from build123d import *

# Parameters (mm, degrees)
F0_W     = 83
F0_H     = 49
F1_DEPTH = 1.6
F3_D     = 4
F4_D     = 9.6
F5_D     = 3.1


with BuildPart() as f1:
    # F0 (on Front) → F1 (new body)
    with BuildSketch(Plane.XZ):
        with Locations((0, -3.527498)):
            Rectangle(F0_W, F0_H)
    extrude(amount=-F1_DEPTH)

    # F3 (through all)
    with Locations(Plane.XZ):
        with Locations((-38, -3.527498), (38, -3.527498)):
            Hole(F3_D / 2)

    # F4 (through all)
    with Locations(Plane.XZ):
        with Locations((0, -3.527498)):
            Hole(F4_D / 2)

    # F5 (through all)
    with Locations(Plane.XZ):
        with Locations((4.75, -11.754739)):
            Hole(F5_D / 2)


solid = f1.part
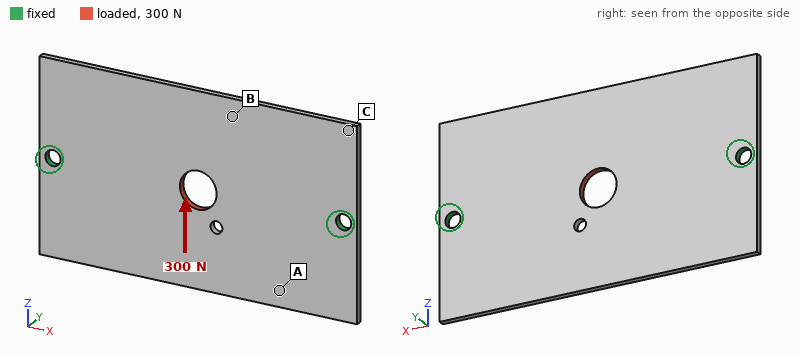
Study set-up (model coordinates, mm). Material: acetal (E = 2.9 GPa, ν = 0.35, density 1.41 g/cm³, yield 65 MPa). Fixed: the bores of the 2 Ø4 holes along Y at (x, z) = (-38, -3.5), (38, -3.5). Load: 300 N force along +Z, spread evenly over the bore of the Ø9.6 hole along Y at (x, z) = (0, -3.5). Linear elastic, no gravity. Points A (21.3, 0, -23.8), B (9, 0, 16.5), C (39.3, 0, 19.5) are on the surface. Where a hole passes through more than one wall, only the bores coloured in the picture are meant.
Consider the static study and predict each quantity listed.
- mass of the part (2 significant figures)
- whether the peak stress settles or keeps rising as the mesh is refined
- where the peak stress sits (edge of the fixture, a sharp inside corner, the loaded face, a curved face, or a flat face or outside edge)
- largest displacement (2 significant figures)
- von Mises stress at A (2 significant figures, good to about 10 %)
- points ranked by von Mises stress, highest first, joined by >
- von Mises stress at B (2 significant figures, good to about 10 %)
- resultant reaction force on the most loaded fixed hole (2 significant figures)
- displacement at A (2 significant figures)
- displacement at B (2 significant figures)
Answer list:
8.9 g
keeps rising
edge of the fixture
0.15 mm
3.6 MPa
B > A > C
6.0 MPa
150 N
0.085 mm
0.12 mm
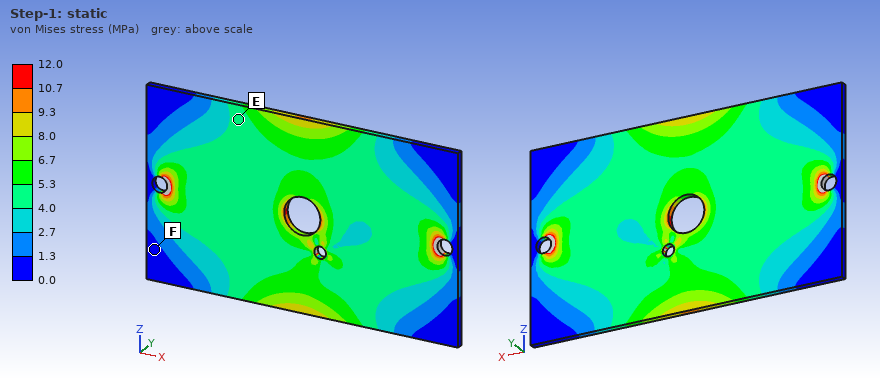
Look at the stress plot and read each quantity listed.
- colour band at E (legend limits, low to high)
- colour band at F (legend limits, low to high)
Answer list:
4.0 to 5.3 MPa
0.0 to 1.3 MPa
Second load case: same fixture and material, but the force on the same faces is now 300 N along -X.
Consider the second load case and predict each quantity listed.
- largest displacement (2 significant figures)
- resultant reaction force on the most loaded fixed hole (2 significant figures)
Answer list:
68 µm
150 N
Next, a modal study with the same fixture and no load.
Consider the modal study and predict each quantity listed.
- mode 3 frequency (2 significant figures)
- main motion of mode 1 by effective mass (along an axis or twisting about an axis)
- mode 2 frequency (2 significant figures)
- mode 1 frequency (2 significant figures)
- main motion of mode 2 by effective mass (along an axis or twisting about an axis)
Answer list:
640 Hz
twisting about X
330 Hz
300 Hz
along Y
